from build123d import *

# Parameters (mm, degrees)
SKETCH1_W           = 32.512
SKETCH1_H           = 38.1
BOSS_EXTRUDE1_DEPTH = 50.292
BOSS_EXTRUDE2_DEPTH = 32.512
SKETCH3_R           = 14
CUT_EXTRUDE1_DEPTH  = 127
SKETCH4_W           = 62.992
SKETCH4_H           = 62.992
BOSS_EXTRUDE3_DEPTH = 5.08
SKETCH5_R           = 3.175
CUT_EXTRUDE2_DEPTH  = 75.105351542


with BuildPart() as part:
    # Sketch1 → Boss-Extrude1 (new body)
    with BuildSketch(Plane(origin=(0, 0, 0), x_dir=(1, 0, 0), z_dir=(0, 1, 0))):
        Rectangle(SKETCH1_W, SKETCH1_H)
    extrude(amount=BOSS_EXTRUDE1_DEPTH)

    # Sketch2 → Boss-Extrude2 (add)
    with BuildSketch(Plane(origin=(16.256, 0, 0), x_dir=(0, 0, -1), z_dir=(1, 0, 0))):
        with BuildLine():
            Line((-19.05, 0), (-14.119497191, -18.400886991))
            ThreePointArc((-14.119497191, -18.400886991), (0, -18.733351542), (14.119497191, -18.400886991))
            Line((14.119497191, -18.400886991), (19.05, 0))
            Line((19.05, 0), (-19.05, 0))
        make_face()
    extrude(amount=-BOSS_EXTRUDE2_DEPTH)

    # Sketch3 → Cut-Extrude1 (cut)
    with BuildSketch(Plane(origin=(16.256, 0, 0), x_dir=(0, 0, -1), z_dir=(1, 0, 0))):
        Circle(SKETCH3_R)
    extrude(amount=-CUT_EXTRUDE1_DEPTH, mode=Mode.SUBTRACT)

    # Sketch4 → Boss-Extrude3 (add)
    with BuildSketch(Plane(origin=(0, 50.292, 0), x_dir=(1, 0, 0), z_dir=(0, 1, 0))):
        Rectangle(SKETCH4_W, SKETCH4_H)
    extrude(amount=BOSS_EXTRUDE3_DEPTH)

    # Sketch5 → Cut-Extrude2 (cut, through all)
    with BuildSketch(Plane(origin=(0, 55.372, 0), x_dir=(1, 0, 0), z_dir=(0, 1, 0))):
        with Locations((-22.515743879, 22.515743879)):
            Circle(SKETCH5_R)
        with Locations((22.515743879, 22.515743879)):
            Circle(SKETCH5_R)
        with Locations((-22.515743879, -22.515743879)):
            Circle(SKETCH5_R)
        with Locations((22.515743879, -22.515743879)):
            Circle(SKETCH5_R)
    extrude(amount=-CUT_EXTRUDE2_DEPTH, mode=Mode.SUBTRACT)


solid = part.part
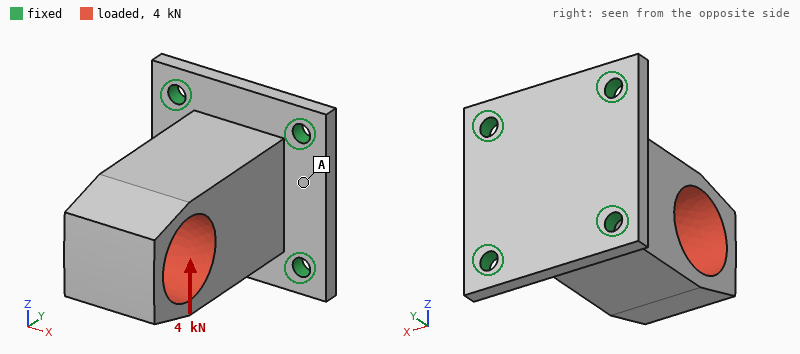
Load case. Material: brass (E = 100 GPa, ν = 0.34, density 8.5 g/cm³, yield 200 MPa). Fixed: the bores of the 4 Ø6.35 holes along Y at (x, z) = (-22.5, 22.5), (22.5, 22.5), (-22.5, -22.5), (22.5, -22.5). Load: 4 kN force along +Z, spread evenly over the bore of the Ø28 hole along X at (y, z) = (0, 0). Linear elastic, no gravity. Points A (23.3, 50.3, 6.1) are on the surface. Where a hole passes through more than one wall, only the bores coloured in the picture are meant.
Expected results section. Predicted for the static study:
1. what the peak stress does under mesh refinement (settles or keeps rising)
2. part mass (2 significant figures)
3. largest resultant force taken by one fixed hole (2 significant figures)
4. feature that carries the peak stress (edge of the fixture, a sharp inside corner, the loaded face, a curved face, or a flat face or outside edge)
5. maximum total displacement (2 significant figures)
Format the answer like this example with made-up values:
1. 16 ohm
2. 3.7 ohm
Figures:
1. keeps rising
2. 700 g
3. 2.9 kN
4. edge of the fixture
5. 0.13 mm
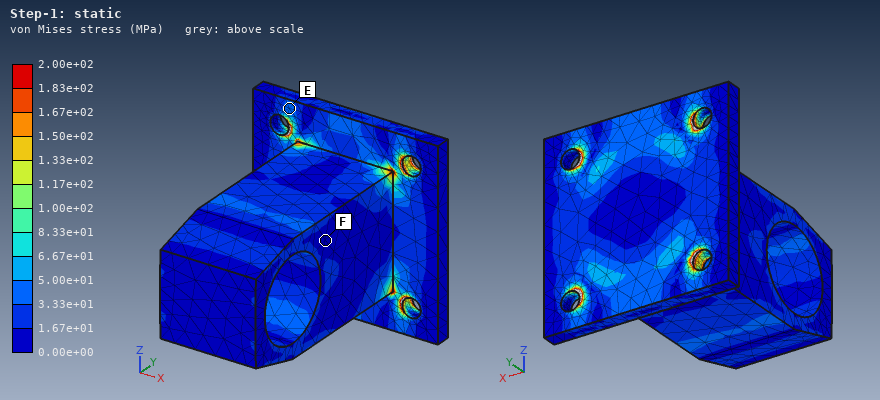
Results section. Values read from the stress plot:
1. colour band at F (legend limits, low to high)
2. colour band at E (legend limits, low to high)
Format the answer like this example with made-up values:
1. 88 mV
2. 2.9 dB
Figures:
1. 0.00e+00 to 1.67e+01 MPa
2. 3.33e+01 to 5.00e+01 MPa
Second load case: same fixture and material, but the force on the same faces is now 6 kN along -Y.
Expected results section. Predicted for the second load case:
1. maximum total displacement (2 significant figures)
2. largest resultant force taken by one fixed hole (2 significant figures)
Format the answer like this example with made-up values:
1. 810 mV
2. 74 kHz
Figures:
1. 24 µm
2. 1.6 kN
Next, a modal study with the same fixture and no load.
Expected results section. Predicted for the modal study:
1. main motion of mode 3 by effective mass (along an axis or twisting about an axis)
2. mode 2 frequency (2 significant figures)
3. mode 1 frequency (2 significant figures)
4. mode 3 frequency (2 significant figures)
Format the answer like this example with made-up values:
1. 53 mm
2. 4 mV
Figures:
1. along Y
2. 2100 Hz
3. 2100 Hz
4. 4300 Hz
